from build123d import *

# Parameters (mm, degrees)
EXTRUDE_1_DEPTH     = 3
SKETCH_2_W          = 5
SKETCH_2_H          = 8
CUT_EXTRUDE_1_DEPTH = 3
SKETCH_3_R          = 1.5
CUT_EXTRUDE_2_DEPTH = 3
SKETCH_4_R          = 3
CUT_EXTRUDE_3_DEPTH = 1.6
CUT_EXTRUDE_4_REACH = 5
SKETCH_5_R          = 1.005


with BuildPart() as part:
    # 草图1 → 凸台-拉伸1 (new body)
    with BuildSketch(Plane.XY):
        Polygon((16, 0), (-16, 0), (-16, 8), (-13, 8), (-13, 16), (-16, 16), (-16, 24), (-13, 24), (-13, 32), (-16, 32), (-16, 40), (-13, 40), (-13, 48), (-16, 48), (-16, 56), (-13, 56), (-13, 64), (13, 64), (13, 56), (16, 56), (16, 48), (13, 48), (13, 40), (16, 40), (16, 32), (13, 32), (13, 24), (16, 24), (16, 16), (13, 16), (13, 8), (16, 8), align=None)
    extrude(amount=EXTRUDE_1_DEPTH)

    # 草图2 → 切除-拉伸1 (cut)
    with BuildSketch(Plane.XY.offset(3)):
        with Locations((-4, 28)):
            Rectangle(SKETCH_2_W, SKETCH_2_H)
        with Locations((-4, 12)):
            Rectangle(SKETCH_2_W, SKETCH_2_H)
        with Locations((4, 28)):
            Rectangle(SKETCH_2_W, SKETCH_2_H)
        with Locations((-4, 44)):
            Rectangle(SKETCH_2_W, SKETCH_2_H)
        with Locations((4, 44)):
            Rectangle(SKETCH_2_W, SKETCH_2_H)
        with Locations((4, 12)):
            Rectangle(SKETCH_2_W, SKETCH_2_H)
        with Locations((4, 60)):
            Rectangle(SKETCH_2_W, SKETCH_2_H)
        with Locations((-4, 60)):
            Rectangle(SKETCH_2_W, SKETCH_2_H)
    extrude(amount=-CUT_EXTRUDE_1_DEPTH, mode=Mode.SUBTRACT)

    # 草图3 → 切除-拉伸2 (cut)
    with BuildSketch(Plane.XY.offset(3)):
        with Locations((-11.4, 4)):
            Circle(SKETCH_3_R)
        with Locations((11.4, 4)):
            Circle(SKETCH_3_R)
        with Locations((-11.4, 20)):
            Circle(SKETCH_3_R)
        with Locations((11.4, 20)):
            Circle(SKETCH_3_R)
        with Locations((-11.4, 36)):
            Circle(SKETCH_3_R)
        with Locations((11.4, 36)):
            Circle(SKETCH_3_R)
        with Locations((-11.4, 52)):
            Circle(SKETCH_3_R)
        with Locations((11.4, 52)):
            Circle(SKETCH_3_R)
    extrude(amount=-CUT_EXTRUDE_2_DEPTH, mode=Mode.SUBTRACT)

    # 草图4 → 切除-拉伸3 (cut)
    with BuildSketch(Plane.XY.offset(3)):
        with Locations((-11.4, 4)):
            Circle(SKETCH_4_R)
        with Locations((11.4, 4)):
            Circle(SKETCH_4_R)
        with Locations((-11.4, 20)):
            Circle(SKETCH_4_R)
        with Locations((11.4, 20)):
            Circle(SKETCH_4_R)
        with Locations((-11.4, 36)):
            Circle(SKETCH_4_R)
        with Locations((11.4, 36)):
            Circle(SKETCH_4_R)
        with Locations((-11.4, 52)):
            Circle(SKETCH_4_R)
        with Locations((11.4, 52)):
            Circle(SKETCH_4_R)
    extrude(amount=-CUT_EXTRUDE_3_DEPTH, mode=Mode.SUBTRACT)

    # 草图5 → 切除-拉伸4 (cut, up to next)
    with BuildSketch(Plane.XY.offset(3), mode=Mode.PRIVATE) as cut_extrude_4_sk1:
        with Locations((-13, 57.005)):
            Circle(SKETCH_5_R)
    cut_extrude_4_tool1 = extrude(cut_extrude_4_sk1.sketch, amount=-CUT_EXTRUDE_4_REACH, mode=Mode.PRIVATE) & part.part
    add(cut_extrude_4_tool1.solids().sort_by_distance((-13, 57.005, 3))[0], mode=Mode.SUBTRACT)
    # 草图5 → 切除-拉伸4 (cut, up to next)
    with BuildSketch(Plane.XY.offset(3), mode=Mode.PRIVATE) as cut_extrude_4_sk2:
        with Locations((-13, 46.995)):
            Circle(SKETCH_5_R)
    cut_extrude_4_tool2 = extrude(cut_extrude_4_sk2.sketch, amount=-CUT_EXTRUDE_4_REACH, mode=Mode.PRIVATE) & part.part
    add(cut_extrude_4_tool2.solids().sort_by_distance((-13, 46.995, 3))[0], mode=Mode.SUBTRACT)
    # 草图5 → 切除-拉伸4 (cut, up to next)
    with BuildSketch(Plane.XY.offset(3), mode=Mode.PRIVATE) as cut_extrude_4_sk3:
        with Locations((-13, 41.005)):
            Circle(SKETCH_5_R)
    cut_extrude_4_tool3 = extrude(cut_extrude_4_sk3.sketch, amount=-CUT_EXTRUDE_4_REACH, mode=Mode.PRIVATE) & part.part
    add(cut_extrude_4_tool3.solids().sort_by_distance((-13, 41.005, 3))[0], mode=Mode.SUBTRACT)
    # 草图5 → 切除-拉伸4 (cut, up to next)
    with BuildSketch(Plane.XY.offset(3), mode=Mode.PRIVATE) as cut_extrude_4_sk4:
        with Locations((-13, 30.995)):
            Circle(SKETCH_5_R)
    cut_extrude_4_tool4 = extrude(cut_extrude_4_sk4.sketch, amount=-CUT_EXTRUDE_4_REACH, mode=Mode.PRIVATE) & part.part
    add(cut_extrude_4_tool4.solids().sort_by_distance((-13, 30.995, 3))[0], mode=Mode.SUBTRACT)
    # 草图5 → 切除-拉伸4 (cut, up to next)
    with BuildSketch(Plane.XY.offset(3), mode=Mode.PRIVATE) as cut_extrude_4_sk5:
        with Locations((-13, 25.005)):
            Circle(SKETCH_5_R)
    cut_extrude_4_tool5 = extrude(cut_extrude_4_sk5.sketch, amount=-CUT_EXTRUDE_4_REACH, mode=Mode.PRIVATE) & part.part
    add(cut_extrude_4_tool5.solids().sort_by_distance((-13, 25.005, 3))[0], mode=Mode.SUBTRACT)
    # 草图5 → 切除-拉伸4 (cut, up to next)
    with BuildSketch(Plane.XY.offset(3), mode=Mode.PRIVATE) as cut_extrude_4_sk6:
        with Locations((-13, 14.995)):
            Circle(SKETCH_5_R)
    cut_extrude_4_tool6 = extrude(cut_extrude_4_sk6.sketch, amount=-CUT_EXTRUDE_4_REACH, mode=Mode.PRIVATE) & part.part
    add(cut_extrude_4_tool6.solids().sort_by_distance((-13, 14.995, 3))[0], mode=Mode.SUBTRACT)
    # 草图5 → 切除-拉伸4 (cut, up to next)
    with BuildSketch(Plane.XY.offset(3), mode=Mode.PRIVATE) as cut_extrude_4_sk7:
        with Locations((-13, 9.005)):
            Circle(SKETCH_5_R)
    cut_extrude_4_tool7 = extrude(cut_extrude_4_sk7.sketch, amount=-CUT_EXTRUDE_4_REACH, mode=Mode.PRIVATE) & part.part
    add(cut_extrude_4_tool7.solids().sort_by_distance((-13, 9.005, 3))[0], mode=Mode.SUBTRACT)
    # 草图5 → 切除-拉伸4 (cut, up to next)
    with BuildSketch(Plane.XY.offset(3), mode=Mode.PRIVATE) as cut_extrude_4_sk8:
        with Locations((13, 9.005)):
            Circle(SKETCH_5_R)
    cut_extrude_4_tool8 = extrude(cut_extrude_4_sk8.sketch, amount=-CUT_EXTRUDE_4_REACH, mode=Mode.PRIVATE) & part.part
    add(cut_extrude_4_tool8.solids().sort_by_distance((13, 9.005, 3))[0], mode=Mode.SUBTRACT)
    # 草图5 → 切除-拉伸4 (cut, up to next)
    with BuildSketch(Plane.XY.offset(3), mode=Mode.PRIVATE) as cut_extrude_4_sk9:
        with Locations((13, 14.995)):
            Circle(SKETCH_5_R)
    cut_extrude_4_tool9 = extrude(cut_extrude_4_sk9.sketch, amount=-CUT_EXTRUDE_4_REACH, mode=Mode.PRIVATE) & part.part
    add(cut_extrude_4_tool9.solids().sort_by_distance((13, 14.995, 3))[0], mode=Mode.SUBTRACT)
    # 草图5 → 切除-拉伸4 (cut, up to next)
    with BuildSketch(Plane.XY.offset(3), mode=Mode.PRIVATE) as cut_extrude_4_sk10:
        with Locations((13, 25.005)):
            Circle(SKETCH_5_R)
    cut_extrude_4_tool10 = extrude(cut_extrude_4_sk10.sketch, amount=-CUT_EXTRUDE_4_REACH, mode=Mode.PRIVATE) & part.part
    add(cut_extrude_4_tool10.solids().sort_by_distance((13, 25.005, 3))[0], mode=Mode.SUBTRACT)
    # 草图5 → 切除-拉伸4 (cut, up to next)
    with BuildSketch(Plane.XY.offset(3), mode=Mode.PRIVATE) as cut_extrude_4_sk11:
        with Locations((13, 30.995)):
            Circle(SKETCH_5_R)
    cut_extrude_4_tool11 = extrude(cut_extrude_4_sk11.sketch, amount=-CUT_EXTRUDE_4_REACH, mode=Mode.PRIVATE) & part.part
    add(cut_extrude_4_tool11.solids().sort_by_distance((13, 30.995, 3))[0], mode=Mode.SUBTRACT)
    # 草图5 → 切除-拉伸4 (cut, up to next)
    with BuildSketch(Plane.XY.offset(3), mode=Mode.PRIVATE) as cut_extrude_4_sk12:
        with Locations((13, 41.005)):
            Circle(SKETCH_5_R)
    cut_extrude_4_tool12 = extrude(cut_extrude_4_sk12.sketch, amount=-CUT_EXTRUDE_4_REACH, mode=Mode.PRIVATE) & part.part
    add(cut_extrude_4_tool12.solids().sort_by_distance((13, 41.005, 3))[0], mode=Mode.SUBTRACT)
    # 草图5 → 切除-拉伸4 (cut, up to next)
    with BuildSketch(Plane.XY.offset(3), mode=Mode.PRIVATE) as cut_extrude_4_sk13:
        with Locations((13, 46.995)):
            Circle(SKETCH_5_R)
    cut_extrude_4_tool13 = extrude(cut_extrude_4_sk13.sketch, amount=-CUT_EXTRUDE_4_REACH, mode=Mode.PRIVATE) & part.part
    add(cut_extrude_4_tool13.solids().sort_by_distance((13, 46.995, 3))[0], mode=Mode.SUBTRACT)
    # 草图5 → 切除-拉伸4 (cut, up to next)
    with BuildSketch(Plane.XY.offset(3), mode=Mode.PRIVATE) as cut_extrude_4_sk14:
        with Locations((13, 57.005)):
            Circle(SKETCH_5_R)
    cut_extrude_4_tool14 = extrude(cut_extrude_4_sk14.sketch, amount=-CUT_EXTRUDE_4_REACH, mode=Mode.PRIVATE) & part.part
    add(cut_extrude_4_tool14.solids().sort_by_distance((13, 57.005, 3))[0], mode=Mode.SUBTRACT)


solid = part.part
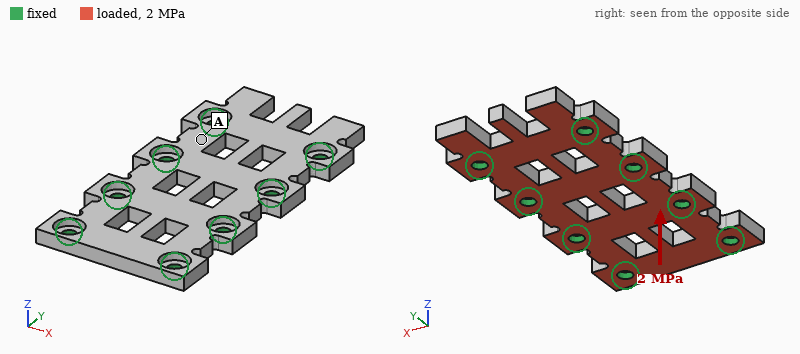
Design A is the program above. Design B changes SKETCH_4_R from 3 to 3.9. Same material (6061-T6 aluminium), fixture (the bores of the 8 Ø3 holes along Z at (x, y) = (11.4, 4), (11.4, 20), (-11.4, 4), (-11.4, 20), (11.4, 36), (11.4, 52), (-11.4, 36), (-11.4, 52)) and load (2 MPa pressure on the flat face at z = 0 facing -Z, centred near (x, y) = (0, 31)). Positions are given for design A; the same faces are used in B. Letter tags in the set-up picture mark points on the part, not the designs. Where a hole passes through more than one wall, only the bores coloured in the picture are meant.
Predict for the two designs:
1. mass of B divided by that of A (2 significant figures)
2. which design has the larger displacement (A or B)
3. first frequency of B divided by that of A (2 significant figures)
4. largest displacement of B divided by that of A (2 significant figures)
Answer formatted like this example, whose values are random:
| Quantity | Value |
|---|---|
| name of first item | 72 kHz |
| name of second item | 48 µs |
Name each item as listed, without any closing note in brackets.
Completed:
| Quantity | Value |
|---|---|
| mass of B divided by that of A | 0.94 |
| which design has the larger displacement | B |
| first frequency of B divided by that of A | 0.89 |
| largest displacement of B divided by that of A | 1.2 |
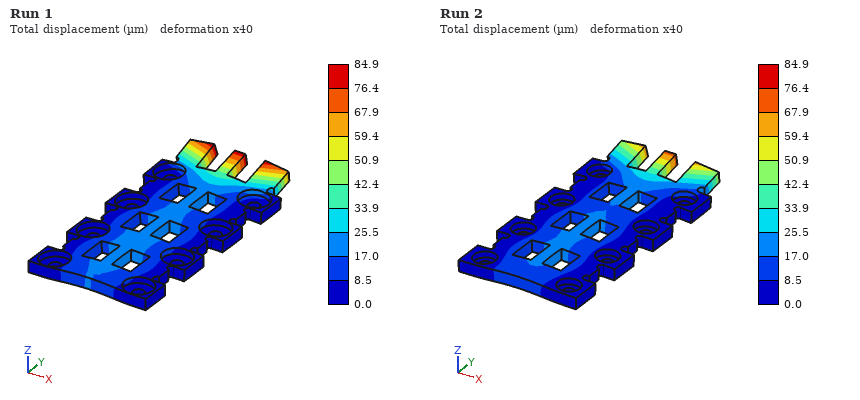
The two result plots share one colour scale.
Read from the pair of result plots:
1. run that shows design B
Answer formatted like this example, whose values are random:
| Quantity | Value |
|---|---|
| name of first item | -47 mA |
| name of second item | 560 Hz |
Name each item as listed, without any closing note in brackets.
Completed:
| Quantity | Value |
|---|---|
| run that shows design B | Run 1 |
